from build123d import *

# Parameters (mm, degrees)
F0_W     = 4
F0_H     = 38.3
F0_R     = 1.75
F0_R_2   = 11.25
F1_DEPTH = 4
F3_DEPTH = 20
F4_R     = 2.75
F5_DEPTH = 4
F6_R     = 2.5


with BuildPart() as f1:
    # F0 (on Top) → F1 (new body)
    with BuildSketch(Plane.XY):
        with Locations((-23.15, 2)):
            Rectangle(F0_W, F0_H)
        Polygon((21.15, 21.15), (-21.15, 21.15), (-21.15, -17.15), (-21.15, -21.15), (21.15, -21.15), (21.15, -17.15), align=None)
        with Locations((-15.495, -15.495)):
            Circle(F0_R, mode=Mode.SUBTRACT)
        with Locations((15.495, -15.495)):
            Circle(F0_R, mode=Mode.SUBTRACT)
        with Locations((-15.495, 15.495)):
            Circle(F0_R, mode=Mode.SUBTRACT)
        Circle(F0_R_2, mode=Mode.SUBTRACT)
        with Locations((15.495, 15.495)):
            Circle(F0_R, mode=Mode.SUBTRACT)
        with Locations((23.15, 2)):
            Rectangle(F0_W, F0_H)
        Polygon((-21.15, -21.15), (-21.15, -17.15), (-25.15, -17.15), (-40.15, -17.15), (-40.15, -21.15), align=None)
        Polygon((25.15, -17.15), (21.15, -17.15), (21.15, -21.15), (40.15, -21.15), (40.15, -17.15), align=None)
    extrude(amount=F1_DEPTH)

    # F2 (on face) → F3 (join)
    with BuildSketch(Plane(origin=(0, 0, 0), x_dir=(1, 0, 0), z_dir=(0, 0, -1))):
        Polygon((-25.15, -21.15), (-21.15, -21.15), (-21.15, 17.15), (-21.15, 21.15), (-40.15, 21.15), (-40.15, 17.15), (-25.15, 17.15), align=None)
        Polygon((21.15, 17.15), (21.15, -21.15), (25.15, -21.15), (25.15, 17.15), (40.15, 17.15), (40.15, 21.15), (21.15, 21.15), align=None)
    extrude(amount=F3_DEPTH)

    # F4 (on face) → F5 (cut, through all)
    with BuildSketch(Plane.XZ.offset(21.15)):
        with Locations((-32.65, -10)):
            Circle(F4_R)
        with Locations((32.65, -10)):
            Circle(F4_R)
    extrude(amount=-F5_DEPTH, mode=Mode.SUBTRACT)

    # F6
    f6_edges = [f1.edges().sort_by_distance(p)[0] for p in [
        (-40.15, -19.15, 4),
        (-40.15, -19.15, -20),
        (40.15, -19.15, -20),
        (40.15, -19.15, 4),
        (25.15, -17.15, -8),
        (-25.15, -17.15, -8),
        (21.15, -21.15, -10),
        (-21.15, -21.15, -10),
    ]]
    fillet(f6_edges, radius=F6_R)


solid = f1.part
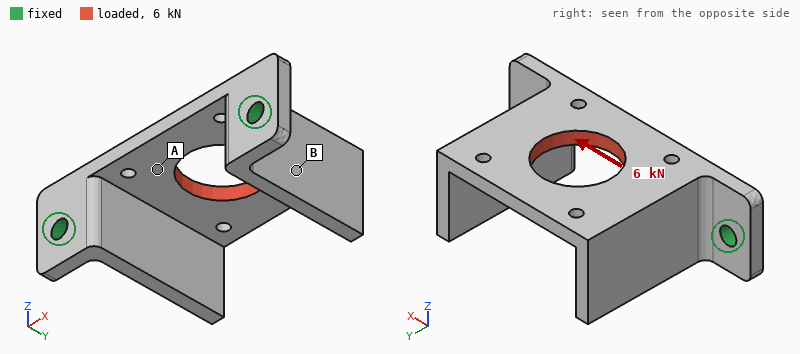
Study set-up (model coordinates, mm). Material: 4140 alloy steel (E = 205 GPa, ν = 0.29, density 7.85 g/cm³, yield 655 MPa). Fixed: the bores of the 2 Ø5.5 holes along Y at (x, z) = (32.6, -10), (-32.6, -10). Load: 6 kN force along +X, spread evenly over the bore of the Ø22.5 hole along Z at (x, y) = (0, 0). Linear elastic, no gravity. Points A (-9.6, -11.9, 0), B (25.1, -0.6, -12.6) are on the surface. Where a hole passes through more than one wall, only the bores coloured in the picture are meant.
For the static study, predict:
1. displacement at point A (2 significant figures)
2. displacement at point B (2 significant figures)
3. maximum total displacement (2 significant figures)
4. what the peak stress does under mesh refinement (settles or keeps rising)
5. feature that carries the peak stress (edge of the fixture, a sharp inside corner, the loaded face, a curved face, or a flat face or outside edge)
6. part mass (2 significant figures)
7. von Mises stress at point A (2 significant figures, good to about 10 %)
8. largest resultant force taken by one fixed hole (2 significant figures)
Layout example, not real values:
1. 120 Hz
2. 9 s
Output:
1. 0.032 mm
2. 0.049 mm
3. 0.11 mm
4. keeps rising
5. edge of the fixture
6. 130 g
7. 86 MPa
8. 3.6 kN
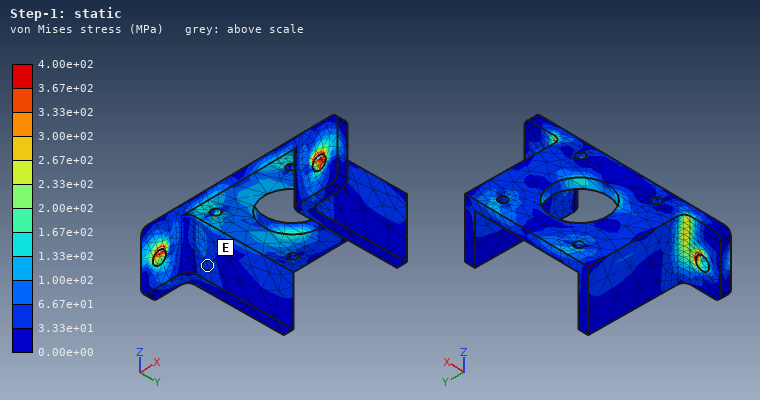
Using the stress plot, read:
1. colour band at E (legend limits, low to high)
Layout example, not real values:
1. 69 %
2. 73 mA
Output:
1. 3.33e+01 to 6.67e+01 MPa
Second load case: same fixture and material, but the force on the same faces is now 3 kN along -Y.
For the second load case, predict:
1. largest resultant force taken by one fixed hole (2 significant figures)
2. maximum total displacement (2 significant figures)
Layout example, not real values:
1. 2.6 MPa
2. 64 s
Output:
1. 1.6 kN
2. 0.12 mm
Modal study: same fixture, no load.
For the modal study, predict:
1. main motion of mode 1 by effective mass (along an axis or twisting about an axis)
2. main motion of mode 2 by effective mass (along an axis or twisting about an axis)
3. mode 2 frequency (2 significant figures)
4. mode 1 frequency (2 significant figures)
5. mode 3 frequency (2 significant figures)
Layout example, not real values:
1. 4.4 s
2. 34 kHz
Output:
1. along Z
2. along X
3. 2800 Hz
4. 2200 Hz
5. 4800 Hz
